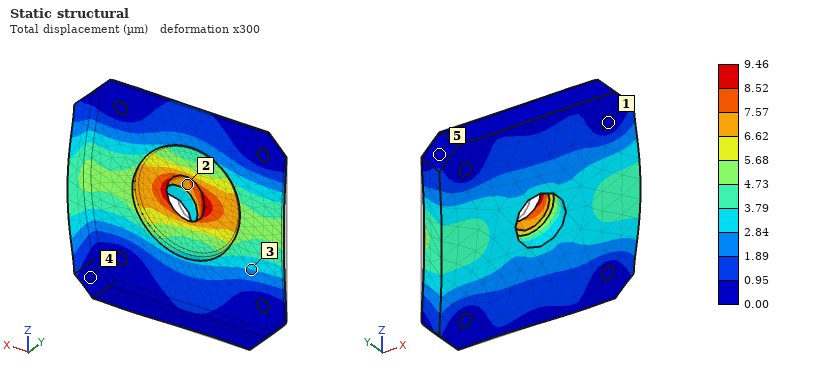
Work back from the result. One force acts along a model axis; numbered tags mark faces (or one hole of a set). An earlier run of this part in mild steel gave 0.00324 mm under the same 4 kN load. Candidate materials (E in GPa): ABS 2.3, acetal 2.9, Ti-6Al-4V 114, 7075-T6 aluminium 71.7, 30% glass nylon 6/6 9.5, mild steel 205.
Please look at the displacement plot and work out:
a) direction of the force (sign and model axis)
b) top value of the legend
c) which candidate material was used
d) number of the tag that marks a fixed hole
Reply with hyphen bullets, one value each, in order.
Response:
- +X
- 9.46 µm
- 7075-T6 aluminium
- 1
